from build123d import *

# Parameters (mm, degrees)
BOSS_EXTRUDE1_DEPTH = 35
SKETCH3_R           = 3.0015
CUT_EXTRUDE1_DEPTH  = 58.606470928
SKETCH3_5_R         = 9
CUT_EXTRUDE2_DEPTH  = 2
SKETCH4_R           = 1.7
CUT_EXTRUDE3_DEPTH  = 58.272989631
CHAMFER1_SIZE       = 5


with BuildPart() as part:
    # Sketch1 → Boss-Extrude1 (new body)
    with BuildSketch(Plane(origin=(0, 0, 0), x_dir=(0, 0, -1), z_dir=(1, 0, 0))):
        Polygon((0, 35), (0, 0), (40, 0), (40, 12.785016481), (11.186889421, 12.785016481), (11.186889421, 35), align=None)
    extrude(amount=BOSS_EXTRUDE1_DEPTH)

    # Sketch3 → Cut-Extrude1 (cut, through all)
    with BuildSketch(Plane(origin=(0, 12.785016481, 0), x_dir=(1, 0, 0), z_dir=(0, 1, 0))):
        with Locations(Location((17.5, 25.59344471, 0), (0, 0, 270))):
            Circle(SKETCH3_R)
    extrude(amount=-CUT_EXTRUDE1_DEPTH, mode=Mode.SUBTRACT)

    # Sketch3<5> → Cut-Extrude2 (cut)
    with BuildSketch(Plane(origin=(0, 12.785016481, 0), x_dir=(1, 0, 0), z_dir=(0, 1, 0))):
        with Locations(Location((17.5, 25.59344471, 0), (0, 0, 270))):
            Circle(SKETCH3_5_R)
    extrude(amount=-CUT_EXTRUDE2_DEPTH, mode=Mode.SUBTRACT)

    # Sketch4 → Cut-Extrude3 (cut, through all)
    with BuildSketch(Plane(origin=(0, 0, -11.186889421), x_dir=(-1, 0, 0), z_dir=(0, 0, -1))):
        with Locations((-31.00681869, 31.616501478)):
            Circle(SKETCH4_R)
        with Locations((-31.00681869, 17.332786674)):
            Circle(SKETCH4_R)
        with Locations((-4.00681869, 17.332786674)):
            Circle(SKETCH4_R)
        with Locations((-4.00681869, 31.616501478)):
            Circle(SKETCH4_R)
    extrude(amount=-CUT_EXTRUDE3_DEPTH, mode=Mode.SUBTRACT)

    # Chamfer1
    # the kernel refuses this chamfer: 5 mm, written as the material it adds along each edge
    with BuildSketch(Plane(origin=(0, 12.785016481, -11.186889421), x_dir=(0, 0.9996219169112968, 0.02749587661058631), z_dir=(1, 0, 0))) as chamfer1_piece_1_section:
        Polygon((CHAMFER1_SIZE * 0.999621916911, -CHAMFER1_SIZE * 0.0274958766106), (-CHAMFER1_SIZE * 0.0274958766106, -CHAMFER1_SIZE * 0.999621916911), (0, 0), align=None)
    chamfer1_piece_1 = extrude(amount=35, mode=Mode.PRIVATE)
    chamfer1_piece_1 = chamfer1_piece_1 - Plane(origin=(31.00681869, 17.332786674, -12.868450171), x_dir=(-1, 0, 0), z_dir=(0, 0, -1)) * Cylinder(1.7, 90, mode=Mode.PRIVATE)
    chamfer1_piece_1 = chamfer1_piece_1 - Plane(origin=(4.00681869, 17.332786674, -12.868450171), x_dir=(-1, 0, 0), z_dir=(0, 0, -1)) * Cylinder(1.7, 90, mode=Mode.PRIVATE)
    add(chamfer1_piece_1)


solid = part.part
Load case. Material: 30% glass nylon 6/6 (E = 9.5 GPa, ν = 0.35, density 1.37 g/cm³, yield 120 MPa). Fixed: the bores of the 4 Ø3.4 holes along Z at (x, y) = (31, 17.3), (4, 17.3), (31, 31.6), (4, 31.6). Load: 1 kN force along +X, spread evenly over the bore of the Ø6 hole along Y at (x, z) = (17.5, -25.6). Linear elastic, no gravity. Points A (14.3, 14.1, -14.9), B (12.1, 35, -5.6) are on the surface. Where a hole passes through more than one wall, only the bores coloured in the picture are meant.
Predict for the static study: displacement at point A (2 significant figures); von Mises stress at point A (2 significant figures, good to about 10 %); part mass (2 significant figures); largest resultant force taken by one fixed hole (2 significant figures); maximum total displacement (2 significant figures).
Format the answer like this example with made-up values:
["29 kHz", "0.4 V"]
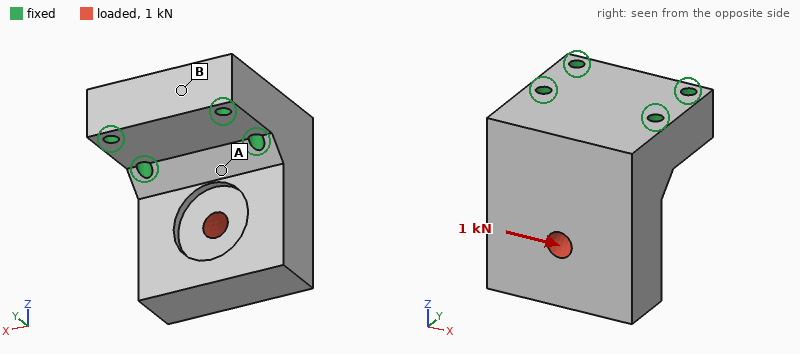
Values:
["11 µm", "9.3 MPa", "35 g", "850 N", "59 µm"]
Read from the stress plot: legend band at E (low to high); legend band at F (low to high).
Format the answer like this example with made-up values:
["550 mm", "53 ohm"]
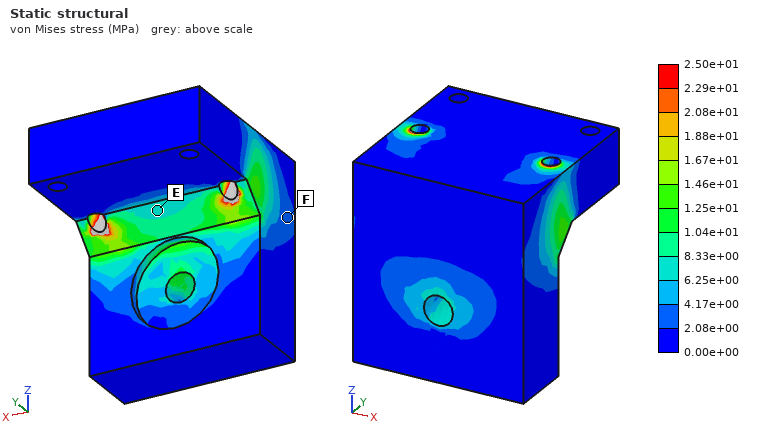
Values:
["6.25e+00 to 8.33e+00 MPa", "2.08e+00 to 4.17e+00 MPa"]
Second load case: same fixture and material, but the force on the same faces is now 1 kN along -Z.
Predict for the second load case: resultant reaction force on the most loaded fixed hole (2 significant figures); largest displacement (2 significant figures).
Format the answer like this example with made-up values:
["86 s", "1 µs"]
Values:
["560 N", "77 µm"]
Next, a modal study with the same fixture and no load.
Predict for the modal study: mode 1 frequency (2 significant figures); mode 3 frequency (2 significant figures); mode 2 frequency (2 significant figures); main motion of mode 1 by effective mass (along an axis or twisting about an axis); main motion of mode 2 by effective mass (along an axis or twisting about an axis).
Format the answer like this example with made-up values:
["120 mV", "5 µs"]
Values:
["3400 Hz", "8500 Hz", "5600 Hz", "along Y", "along X"]
